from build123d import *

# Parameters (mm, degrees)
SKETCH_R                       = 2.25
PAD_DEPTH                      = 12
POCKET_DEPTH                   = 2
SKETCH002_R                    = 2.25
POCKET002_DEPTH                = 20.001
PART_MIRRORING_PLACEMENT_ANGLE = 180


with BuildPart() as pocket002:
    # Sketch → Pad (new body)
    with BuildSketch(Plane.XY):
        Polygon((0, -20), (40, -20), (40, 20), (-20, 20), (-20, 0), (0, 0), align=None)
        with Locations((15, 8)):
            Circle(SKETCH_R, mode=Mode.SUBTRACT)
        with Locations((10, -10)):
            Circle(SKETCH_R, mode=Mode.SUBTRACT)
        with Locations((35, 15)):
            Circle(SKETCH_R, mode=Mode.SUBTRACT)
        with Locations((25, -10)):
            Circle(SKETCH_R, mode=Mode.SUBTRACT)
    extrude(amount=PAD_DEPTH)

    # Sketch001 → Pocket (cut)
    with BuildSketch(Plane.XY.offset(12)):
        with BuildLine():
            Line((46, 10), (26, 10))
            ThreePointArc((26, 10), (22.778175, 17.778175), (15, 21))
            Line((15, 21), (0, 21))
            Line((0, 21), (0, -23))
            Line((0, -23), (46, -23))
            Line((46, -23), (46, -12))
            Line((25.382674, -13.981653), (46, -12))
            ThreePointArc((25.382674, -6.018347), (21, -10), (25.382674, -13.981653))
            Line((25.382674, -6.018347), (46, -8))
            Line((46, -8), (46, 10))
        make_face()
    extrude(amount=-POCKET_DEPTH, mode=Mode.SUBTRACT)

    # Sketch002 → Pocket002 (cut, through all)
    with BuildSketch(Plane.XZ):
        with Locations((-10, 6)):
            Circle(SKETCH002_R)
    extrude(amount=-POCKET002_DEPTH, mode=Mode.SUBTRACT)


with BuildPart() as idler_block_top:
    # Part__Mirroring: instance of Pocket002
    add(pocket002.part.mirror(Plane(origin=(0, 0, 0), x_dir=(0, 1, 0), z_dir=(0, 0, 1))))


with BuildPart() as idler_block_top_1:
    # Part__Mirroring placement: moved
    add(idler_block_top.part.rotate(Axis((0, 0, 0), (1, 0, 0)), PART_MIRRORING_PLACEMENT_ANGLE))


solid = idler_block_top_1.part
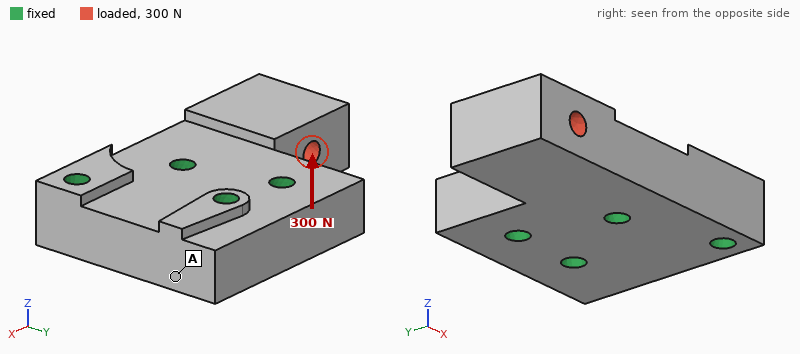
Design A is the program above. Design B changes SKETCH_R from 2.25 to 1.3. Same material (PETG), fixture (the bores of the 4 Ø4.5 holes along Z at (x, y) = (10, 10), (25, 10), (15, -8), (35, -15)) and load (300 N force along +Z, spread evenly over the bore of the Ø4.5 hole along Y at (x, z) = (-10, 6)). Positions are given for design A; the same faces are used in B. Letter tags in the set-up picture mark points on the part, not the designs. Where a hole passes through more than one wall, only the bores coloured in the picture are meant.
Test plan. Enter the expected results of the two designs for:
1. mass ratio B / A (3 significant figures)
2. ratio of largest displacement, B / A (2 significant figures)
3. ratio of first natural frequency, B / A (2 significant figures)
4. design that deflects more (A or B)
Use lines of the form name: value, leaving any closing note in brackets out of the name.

mass ratio B / A: 1.02
ratio of largest displacement, B / A: 1.1
ratio of first natural frequency, B / A: 0.94
design that deflects more: B
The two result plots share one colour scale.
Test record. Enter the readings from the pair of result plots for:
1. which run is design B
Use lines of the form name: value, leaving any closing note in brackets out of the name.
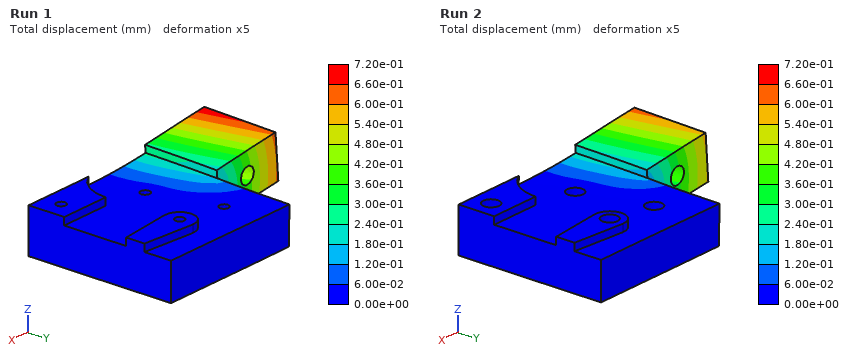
which run is design B: Run 1
